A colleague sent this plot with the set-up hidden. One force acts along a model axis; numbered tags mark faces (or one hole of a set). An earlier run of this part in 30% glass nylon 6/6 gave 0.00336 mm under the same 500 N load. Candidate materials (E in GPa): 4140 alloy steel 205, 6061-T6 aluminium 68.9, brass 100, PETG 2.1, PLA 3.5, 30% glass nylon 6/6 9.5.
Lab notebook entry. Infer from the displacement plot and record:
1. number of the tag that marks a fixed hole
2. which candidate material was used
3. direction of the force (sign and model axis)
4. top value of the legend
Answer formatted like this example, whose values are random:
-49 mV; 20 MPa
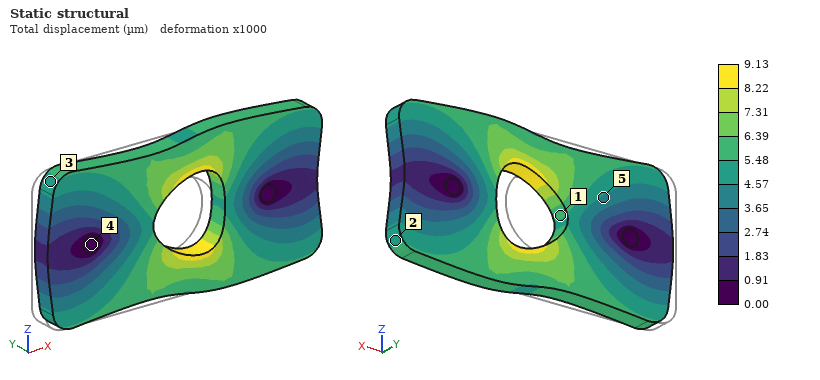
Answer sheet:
4; PLA; +X; 9.13 µm
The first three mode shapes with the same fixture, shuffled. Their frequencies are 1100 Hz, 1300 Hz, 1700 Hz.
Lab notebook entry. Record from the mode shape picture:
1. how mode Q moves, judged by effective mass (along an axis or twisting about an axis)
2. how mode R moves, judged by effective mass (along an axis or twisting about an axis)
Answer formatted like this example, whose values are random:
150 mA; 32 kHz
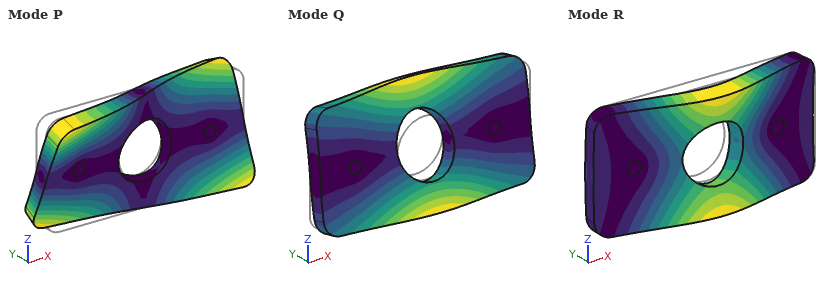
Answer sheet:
twisting about X; along Y
